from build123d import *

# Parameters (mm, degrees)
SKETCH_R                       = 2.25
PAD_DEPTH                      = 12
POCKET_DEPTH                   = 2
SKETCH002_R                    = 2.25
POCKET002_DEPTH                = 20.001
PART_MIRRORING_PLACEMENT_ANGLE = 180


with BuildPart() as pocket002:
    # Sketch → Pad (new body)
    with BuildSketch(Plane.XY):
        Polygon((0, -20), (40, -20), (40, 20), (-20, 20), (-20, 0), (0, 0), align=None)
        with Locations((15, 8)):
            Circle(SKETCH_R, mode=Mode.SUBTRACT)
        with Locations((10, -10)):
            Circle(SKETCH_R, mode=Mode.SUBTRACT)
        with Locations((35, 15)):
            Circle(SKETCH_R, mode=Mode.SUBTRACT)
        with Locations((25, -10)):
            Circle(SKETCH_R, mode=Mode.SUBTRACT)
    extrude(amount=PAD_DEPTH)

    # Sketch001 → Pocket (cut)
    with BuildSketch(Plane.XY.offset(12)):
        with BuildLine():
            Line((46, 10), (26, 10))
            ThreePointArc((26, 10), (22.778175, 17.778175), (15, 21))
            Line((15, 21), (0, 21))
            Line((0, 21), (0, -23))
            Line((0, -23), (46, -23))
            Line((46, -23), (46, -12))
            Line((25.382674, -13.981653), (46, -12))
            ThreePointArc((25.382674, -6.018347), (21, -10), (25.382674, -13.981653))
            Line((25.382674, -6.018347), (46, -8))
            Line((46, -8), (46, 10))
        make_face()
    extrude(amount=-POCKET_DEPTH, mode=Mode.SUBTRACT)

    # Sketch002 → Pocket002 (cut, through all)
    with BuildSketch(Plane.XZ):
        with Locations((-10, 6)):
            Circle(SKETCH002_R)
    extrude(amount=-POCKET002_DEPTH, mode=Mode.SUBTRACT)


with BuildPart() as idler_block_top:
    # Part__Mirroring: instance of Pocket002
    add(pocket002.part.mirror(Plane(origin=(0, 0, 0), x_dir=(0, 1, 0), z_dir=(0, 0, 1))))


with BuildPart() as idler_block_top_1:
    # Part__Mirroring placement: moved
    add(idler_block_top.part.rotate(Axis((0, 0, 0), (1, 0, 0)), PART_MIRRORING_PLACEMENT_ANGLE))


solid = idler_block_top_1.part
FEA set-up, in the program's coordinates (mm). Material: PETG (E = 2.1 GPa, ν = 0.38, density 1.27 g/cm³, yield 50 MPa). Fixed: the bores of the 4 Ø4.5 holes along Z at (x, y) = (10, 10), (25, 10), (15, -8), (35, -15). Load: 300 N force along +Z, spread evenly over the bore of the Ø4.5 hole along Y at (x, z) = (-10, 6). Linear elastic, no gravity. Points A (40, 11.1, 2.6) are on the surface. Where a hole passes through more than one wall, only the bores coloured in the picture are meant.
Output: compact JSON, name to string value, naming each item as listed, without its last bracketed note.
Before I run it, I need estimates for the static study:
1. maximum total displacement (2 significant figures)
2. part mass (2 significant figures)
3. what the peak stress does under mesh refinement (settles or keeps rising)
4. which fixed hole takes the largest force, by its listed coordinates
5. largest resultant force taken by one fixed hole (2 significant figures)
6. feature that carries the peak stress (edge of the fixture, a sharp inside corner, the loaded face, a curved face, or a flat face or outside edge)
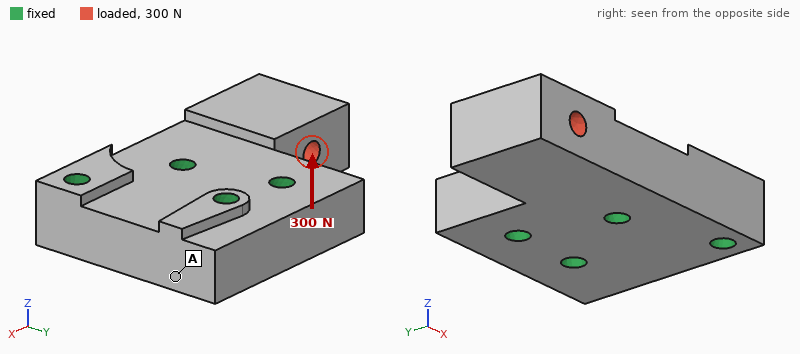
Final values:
{"maximum total displacement": "0.64 mm", "part mass": "26 g", "what the peak stress does under mesh refinement": "keeps rising", "which fixed hole takes the largest force, by its listed coordinates": "(15, -8)", "largest resultant force taken by one fixed hole": "300 N", "feature that carries the peak stress": "edge of the fixture"}
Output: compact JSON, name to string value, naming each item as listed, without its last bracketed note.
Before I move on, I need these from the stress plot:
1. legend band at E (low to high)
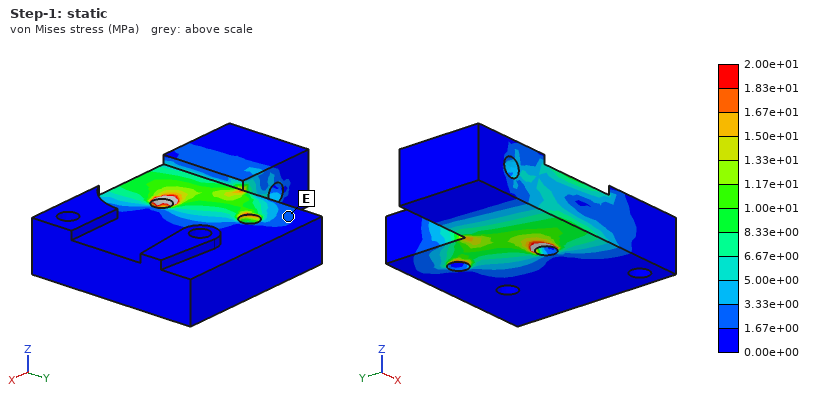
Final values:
{"legend band at E": "1.67e+00 to 3.33e+00 MPa"}
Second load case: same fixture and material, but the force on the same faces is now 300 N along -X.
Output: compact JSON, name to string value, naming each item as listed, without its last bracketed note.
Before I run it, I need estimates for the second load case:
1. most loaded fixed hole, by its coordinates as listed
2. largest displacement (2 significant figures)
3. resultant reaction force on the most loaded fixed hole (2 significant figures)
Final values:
{"most loaded fixed hole, by its coordinates as listed": "(15, -8)", "largest displacement": "49 µm", "resultant reaction force on the most loaded fixed hole": "220 N"}
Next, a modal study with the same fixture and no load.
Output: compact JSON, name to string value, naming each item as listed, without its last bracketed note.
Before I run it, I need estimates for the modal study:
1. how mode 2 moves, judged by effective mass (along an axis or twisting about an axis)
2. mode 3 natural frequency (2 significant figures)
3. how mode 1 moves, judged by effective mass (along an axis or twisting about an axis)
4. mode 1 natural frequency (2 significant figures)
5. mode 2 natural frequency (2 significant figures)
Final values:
{"how mode 2 moves, judged by effective mass": "along Y", "mode 3 natural frequency": "4700 Hz", "how mode 1 moves, judged by effective mass": "along Z", "mode 1 natural frequency": "1700 Hz", "mode 2 natural frequency": "3400 Hz"}
